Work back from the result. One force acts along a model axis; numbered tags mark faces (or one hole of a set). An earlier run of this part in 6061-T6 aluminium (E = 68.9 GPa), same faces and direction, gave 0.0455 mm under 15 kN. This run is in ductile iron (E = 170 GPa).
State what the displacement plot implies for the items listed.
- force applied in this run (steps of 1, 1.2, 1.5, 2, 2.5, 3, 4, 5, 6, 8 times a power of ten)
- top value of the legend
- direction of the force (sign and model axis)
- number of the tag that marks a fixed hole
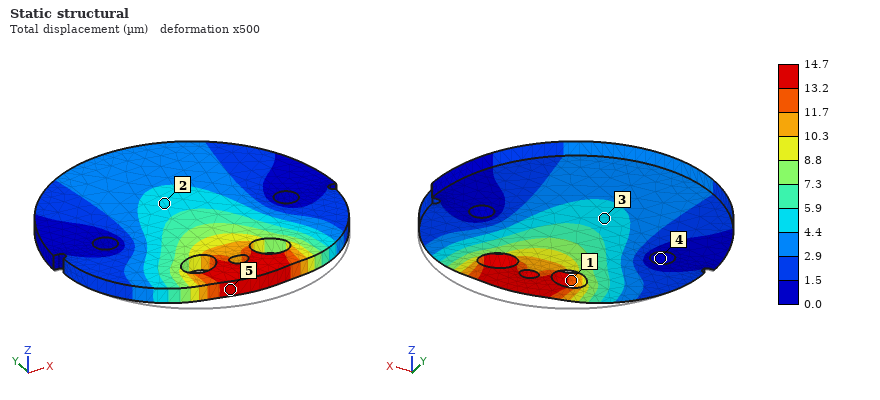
12 kN
14.7 µm
+Y
4
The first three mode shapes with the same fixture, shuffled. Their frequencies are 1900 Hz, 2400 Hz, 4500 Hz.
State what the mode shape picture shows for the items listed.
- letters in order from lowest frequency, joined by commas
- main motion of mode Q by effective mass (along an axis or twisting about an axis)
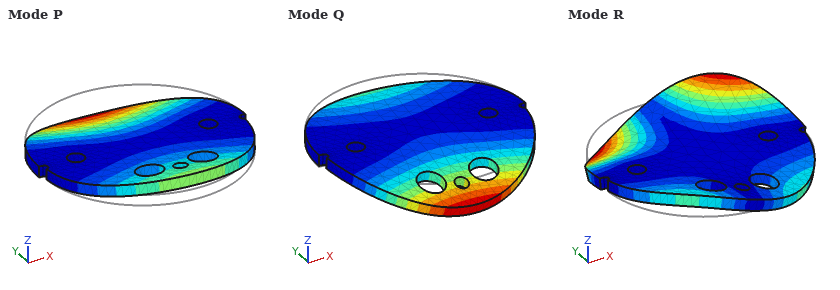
P, Q, R
along Z
